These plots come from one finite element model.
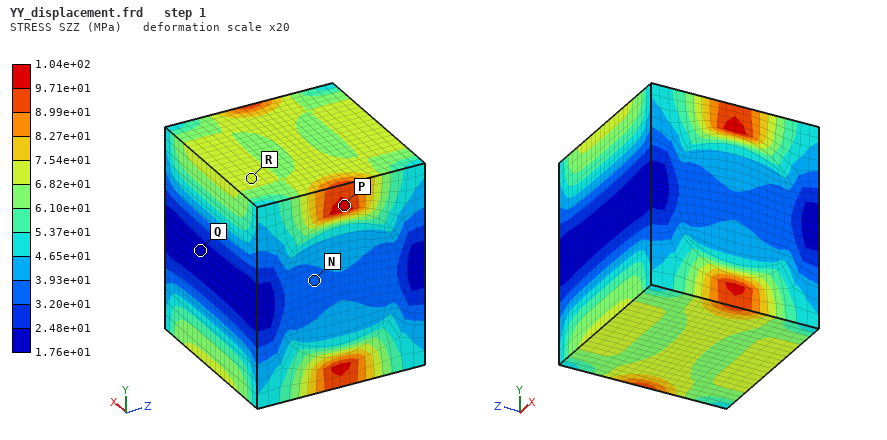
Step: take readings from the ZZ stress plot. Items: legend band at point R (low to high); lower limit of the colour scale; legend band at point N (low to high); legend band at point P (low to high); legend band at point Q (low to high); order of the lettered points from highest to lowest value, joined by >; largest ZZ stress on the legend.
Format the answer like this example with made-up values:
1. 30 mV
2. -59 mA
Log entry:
1. 6.82e+01 to 7.54e+01 MPa
2. 1.76e+01 MPa
3. 3.20e+01 to 3.93e+01 MPa
4. 9.71e+01 to 1.04e+02 MPa
5. 1.76e+01 to 2.48e+01 MPa
6. P > R > N > Q
7. 1.04e+02 MPa
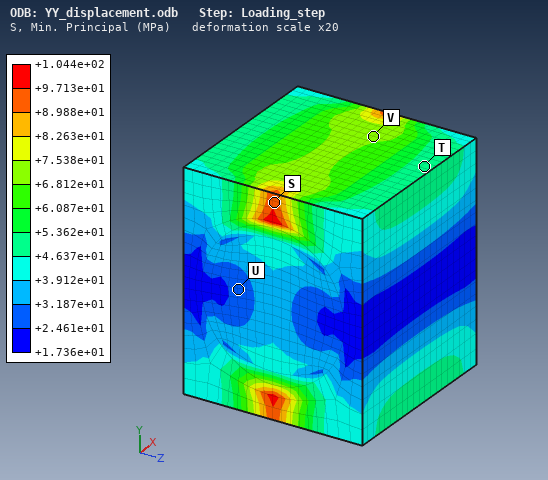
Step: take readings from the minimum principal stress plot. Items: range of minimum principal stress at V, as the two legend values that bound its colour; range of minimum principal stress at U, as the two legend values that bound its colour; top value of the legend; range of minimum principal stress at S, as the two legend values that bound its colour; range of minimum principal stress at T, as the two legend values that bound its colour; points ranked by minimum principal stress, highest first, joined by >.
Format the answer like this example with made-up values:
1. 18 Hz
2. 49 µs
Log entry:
1. +6.812e+01 to +7.538e+01 MPa
2. +2.461e+01 to +3.187e+01 MPa
3. +1.044e+02 MPa
4. +8.988e+01 to +9.713e+01 MPa
5. +4.637e+01 to +5.362e+01 MPa
6. S > V > T > U
